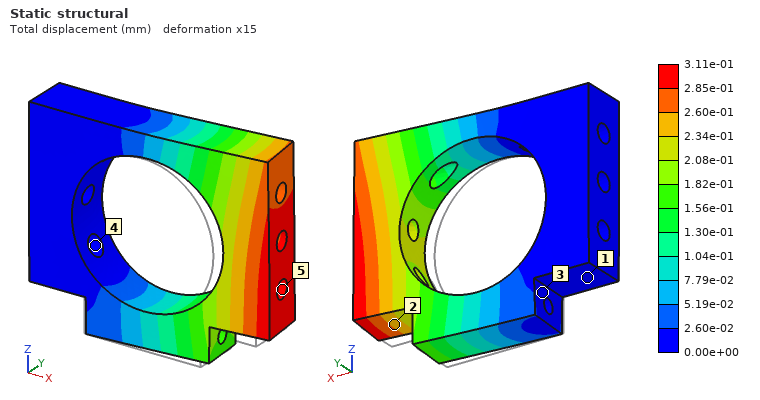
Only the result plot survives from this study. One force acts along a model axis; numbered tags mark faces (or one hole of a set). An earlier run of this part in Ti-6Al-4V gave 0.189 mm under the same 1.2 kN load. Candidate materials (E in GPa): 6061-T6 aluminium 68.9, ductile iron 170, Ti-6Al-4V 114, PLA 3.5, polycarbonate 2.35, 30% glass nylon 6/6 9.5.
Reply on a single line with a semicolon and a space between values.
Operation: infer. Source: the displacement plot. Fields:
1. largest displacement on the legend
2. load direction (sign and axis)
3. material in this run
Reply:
3.11e-01 mm; +Y; 6061-T6 aluminium
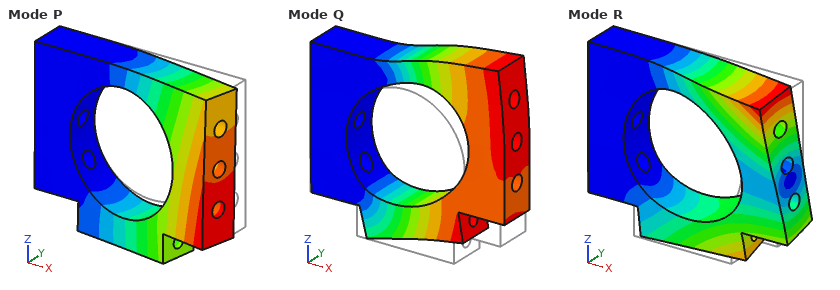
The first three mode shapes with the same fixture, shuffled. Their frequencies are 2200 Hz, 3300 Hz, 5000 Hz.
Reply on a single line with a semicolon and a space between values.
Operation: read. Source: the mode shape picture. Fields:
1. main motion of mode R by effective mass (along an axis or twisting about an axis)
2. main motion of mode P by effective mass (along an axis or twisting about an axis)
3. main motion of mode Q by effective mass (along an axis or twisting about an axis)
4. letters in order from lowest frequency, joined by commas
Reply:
twisting about X; along Y; along Z; P, Q, R
